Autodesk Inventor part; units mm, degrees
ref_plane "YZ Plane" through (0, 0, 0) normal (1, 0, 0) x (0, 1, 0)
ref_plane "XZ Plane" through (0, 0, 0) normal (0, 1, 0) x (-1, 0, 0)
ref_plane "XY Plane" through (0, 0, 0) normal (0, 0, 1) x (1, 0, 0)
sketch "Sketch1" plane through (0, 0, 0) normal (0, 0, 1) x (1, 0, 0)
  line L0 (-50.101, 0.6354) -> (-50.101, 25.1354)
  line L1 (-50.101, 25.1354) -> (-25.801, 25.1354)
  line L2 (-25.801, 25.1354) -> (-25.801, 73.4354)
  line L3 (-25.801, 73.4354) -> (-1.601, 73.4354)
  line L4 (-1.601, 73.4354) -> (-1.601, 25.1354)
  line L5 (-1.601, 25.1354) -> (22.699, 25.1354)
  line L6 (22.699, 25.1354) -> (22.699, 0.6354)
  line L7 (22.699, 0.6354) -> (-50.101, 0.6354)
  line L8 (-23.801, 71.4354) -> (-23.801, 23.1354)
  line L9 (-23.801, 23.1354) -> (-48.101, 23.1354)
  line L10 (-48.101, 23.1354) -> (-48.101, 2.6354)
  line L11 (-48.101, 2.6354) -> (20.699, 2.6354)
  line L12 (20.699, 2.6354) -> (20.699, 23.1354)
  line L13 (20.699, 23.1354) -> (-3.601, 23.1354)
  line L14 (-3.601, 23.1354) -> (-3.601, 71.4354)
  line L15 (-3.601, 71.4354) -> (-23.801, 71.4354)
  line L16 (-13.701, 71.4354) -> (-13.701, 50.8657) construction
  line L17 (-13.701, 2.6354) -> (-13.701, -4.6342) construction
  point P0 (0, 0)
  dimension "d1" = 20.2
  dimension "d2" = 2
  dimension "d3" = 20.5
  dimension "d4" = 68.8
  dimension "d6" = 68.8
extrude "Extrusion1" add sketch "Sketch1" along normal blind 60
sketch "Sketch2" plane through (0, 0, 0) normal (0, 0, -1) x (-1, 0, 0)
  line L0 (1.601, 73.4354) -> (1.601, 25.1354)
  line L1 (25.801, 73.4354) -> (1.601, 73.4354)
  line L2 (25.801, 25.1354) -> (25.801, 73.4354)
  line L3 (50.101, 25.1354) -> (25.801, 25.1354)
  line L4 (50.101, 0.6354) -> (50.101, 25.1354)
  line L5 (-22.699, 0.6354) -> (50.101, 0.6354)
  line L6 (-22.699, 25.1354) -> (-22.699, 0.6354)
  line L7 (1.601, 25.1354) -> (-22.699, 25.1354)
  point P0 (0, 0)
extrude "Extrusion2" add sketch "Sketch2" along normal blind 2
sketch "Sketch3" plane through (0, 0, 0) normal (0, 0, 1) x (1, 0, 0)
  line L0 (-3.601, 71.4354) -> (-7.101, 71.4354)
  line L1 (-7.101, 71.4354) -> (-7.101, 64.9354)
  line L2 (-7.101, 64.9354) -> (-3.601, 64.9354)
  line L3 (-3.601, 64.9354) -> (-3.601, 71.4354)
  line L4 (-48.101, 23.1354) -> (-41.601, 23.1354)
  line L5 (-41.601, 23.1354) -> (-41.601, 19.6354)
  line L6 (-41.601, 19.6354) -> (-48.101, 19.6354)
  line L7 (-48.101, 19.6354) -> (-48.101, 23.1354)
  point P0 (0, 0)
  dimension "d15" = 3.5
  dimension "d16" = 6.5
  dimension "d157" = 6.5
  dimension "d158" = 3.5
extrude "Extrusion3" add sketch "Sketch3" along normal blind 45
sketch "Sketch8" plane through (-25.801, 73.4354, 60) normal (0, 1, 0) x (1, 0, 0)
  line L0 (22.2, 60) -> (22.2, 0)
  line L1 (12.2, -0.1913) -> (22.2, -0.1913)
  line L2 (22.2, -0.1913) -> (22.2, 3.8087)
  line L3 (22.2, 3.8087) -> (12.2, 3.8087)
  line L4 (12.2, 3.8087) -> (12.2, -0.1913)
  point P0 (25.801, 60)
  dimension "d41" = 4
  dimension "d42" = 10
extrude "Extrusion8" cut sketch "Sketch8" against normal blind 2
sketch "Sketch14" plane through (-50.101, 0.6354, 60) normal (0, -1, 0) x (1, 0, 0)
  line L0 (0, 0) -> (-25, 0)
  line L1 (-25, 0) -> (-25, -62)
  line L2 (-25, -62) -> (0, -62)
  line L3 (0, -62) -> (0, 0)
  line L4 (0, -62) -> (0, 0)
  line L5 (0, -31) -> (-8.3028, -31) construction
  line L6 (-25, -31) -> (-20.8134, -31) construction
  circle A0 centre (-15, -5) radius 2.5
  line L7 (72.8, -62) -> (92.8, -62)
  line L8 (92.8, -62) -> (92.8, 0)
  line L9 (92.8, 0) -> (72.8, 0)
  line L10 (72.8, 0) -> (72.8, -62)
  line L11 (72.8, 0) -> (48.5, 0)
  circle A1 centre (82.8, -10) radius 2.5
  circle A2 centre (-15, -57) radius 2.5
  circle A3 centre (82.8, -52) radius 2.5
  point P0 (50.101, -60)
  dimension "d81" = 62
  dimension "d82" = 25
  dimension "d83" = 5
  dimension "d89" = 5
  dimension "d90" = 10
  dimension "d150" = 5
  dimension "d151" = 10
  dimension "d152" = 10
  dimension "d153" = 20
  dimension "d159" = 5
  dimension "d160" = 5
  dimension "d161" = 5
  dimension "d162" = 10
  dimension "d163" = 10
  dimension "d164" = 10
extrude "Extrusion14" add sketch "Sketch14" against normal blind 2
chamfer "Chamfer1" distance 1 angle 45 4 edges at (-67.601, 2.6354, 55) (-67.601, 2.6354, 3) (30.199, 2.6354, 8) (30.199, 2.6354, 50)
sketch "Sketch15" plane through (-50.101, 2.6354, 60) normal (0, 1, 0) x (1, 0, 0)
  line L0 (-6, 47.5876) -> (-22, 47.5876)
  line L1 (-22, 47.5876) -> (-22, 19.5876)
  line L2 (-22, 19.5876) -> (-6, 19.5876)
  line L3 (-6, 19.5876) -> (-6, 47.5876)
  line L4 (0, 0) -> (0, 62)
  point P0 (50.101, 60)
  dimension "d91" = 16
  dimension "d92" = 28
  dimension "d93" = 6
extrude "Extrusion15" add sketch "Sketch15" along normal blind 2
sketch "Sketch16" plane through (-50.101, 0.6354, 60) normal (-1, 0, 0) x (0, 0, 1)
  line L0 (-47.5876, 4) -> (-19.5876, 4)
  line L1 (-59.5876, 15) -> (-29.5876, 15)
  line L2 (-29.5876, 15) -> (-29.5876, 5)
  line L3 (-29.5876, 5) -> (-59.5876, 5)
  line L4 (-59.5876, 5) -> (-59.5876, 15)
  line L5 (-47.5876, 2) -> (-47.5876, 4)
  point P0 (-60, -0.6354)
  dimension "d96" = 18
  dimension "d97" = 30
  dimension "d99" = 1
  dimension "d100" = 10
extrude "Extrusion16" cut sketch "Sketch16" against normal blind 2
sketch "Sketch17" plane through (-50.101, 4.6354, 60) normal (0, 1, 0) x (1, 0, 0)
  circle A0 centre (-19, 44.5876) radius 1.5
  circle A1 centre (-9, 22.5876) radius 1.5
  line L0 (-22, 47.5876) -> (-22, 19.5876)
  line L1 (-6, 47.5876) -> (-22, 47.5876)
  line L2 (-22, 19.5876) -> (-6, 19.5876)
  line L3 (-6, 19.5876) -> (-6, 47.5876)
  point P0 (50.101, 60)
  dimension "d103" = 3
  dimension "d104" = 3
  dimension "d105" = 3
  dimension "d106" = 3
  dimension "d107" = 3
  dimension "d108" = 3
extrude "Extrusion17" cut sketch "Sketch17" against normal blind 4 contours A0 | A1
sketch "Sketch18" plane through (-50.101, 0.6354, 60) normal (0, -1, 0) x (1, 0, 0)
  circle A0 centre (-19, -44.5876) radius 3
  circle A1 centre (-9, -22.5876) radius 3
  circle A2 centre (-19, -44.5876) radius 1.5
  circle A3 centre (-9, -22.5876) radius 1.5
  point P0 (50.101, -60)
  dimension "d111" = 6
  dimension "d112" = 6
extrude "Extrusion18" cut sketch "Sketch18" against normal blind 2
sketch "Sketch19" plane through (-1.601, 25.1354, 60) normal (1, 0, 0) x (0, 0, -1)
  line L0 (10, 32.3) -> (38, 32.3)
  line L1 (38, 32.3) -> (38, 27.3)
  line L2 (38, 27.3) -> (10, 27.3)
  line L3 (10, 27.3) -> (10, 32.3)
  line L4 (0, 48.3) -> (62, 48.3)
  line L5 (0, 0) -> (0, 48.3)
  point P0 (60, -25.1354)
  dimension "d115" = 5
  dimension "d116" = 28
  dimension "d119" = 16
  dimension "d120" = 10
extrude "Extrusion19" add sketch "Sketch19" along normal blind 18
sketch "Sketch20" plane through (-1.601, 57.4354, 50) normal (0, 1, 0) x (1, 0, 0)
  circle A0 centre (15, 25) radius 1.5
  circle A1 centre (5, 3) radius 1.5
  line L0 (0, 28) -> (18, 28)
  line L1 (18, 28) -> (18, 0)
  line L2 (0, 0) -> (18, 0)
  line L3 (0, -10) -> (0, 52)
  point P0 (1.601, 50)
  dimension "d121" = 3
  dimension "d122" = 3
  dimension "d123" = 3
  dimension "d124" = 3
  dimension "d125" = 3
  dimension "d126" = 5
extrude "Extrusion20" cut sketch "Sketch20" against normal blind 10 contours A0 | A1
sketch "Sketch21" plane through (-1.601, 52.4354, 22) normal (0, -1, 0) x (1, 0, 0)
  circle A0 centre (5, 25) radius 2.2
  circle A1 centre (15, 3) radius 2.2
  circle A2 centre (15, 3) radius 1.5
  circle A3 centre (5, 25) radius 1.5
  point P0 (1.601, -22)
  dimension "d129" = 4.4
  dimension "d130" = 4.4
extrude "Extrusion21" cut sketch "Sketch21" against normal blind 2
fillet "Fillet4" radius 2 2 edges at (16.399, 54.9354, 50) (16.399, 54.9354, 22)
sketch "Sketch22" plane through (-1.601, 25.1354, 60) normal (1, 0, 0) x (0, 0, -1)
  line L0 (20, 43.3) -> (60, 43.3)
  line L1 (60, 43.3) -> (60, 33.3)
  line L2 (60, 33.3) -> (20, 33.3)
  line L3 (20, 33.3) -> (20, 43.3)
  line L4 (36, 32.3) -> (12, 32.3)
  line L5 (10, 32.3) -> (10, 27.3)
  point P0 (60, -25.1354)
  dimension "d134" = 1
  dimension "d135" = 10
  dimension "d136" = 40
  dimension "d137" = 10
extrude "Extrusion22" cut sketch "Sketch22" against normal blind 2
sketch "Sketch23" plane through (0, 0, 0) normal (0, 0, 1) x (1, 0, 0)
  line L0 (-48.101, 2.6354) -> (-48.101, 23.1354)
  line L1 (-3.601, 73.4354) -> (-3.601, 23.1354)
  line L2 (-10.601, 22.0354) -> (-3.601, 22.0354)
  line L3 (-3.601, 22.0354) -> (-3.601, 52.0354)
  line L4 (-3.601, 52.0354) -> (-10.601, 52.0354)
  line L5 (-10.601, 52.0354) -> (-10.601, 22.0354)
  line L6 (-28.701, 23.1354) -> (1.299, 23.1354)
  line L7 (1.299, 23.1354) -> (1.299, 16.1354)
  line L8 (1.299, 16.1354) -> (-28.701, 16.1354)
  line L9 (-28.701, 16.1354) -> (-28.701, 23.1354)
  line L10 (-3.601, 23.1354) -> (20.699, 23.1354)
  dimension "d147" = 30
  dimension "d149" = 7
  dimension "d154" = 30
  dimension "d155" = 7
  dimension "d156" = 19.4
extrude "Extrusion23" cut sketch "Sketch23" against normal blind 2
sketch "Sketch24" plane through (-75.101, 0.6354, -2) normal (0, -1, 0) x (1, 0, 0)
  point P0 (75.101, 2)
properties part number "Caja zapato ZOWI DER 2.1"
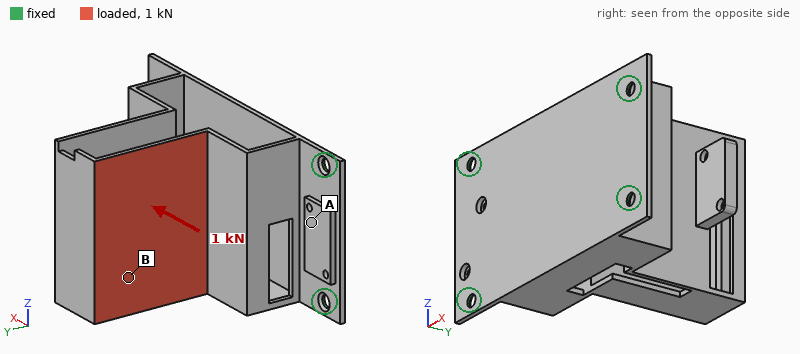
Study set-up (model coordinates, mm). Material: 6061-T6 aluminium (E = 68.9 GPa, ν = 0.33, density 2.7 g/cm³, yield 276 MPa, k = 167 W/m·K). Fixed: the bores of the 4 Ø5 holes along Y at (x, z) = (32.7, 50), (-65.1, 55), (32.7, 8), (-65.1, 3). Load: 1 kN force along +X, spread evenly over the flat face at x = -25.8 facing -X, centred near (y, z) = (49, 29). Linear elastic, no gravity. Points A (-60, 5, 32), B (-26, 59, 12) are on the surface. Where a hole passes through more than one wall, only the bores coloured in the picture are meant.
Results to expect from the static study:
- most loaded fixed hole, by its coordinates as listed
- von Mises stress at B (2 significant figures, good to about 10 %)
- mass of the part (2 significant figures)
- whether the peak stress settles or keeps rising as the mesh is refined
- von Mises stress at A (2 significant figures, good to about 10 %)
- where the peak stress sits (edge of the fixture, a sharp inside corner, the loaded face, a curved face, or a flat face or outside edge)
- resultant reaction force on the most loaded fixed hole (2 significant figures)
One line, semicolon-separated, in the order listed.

(32.7, 8); 32 MPa; 130 g; keeps rising; 18 MPa; edge of the fixture; 610 N
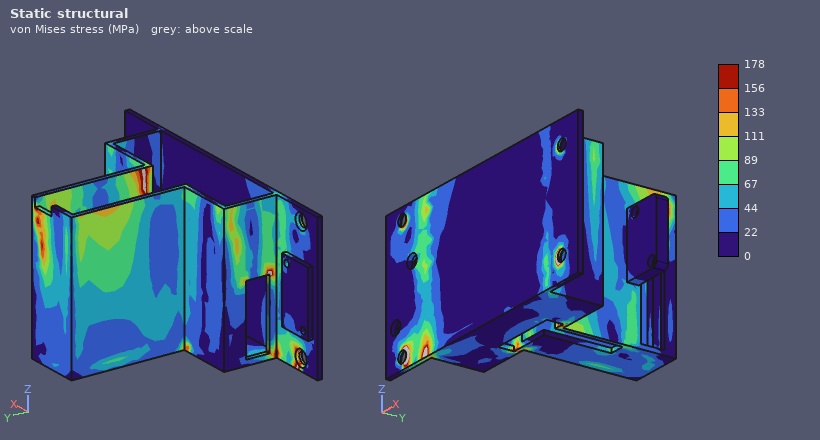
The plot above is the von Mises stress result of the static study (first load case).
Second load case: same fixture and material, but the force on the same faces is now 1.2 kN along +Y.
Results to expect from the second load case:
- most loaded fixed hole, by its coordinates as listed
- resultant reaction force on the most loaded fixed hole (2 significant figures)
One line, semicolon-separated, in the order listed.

(-65.1, 3); 860 N
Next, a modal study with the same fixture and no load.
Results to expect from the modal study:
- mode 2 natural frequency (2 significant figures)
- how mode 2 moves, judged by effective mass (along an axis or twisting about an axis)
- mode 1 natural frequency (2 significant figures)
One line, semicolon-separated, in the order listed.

720 Hz; along X; 640 Hz
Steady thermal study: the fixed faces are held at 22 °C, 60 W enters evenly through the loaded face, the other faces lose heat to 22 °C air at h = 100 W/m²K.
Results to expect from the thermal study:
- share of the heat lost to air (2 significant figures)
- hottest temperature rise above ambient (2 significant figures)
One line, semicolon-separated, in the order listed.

89 %; 50 K
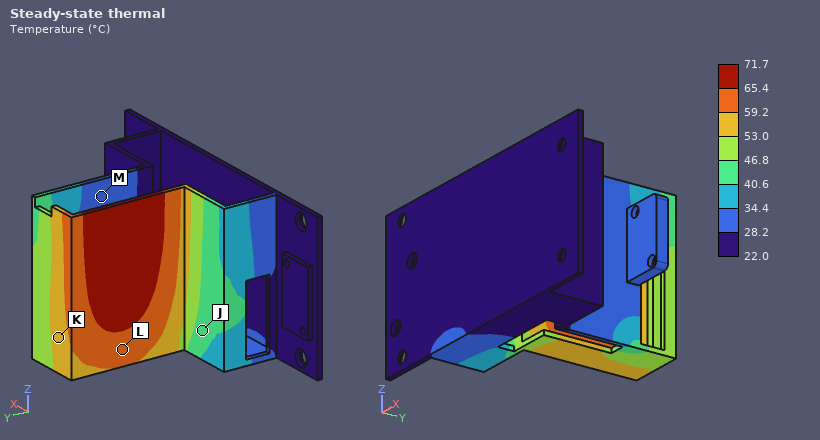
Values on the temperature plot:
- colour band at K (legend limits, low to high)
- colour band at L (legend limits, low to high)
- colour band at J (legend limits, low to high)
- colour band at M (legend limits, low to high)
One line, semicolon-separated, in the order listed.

53.0 to 59.2 °C; 59.2 to 65.4 °C; 40.6 to 46.8 °C; 28.2 to 34.4 °C
